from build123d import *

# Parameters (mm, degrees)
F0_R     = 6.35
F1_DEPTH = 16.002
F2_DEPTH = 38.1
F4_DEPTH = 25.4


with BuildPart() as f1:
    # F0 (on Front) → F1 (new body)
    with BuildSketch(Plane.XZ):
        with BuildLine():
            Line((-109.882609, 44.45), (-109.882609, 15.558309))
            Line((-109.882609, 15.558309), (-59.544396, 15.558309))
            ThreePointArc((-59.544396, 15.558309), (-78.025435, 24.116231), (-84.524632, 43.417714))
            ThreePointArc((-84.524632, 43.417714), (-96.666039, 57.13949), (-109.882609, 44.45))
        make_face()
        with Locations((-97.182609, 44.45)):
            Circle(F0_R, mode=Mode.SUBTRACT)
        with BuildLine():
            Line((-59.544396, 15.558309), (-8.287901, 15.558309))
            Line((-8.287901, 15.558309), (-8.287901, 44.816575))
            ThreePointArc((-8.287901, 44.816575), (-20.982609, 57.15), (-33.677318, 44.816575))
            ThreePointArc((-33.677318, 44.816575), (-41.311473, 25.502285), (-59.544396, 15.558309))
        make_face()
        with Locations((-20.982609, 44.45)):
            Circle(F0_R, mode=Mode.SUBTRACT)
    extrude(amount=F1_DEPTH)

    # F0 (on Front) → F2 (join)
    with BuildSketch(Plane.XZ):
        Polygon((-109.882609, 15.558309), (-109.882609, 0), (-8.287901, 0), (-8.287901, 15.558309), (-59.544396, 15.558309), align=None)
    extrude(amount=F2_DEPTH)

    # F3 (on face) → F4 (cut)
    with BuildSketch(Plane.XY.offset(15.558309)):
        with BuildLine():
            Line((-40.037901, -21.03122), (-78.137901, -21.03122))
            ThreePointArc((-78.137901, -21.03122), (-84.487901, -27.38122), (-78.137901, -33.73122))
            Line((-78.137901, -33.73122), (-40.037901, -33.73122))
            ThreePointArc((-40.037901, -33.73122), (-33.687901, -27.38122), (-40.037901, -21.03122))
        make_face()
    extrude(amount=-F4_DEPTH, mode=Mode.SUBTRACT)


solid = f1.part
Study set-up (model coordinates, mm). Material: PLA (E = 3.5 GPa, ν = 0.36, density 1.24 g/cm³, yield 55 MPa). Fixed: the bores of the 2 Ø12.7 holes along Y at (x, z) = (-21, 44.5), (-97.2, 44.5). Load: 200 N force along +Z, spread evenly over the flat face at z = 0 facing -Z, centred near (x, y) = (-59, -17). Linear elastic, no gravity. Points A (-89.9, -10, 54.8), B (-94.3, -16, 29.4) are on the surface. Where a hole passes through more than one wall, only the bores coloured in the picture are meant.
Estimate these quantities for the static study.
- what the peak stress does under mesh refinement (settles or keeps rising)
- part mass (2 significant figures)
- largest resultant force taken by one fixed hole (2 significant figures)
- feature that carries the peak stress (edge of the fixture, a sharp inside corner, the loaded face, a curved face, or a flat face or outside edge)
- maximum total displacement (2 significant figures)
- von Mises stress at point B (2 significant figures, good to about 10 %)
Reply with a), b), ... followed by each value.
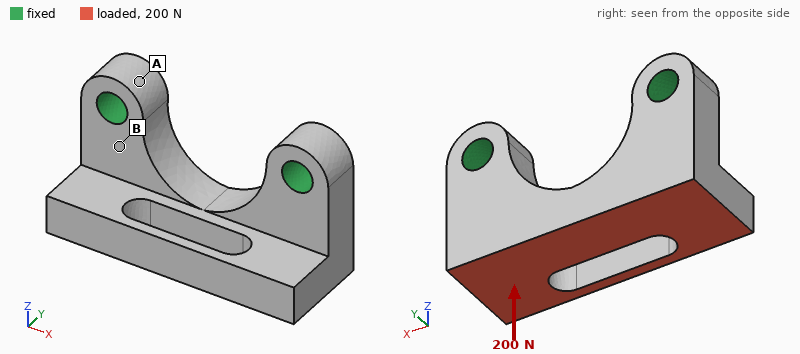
a) keeps rising
b) 100 g
c) 100 N
d) edge of the fixture
e) 43 µm
f) 1.1 MPa
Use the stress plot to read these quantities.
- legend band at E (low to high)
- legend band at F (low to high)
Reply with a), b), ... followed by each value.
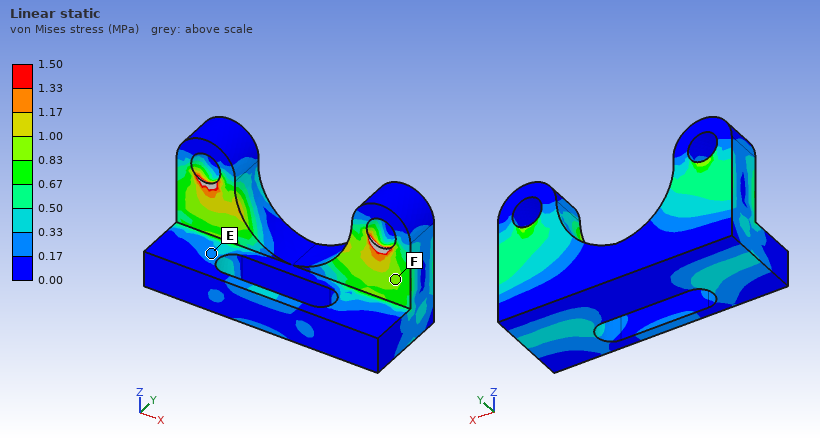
a) 0.17 to 0.33 MPa
b) 0.83 to 1.00 MPa
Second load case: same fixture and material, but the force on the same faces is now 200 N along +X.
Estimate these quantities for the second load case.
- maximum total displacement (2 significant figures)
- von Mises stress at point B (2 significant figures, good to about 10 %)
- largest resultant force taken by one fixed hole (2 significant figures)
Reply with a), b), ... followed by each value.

a) 21 µm
b) 0.69 MPa
c) 130 N
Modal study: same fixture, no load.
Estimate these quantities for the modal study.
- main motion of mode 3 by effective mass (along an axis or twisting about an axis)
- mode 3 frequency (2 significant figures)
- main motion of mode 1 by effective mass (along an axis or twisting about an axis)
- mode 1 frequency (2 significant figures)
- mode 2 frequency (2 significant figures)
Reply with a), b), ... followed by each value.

a) along X
b) 2500 Hz
c) along Y
d) 1100 Hz
e) 1700 Hz
